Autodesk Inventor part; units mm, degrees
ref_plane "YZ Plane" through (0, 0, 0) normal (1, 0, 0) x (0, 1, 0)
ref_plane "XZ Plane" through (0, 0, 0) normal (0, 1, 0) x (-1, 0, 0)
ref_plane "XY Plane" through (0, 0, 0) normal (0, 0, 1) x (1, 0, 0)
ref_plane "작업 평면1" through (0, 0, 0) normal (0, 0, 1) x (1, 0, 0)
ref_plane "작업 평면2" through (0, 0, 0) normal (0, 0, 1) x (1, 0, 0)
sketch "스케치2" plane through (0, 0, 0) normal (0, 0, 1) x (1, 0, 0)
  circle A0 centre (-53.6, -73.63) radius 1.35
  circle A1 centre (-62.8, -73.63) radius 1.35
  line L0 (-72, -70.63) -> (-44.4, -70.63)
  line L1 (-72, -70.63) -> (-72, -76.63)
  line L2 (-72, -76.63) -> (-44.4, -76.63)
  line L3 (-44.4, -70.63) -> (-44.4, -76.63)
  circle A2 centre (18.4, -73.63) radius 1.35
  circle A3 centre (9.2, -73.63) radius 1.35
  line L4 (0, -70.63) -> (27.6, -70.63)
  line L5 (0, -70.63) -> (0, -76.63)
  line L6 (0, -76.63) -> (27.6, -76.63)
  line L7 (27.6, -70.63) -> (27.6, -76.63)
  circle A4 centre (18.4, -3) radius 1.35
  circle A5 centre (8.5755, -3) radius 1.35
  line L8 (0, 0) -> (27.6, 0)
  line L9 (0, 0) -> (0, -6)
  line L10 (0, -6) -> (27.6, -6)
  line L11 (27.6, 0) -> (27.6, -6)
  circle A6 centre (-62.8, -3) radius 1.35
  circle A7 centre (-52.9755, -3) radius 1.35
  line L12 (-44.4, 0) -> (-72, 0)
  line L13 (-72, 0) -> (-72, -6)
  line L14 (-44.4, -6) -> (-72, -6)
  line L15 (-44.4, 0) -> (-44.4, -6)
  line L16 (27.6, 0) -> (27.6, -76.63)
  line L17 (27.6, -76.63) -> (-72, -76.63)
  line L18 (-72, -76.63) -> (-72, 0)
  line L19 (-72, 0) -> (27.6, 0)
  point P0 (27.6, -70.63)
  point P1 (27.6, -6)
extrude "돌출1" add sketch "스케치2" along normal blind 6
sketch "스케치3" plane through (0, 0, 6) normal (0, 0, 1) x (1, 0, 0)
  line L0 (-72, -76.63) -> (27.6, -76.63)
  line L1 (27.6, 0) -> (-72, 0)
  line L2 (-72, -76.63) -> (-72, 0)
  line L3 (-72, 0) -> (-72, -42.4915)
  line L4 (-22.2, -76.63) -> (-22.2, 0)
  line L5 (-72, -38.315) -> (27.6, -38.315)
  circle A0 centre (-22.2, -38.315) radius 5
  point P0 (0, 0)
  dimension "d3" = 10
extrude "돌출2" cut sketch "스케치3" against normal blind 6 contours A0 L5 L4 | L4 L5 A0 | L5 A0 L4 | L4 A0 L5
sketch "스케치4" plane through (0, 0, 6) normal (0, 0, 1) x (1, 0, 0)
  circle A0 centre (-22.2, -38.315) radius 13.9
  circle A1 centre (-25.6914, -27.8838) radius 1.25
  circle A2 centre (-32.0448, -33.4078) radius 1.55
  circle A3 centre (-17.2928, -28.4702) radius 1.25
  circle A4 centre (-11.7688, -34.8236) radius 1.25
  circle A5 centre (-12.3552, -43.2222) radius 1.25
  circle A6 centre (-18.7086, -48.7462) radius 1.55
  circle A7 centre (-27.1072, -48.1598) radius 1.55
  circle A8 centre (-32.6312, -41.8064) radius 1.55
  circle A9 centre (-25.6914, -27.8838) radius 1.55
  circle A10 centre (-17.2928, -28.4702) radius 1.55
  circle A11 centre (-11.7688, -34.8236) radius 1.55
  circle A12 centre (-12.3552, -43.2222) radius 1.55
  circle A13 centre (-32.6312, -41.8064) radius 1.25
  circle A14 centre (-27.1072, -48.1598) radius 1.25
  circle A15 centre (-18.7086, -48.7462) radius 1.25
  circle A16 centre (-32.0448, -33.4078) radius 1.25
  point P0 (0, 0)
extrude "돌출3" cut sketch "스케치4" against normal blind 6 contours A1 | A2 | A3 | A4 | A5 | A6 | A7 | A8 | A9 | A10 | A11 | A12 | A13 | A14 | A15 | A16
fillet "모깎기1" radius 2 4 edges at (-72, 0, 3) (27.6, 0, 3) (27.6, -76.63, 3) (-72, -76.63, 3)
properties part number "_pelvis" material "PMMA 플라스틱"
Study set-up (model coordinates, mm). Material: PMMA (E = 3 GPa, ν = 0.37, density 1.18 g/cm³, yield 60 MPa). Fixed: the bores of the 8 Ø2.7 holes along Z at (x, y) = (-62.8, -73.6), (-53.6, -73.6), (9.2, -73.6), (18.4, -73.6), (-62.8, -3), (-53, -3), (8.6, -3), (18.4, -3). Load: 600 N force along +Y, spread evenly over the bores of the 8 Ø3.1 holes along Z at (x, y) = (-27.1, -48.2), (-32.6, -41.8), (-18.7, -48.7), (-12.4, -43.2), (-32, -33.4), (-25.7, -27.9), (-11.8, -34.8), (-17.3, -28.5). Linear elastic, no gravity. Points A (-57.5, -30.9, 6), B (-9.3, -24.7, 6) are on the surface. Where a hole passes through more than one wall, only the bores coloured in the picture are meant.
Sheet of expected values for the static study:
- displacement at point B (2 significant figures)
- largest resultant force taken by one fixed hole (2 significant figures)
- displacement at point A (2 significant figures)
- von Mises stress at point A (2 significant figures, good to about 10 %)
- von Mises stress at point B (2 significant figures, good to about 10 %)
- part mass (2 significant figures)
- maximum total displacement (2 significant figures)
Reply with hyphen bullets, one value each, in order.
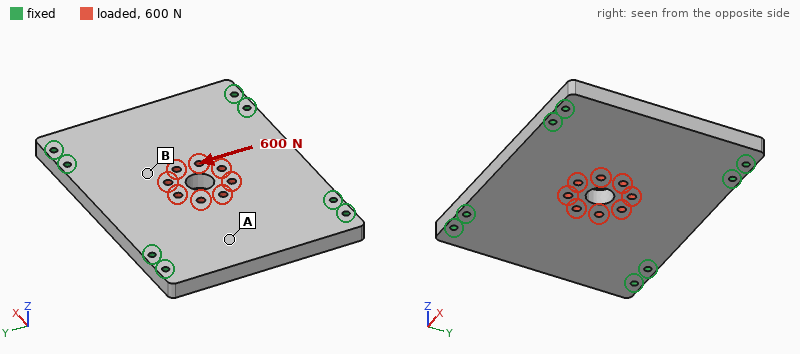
- 18 µm
- 120 N
- 6.3 µm
- 0.46 MPa
- 1.4 MPa
- 53 g
- 26 µm
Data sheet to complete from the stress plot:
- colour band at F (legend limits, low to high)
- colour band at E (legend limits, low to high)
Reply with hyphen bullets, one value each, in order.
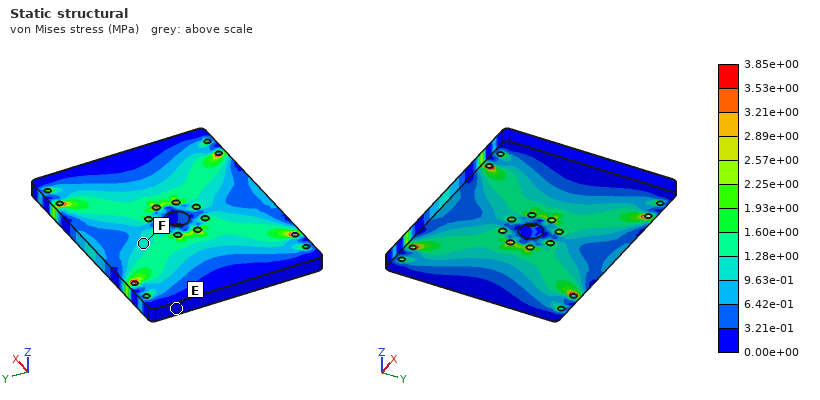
- 9.63e-01 to 1.28e+00 MPa
- 0.00e+00 to 3.21e-01 MPa
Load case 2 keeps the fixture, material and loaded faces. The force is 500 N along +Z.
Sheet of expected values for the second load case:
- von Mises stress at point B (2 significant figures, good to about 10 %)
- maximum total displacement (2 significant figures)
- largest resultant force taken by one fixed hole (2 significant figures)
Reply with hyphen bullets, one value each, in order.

- 7.2 MPa
- 0.62 mm
- 160 N
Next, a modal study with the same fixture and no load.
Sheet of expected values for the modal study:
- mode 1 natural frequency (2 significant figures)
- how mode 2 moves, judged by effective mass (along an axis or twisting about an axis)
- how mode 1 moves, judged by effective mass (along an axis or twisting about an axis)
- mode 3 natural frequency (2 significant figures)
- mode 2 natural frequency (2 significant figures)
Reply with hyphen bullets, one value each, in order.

- 1300 Hz
- twisting about Y
- along Z
- 2100 Hz
- 1900 Hz
